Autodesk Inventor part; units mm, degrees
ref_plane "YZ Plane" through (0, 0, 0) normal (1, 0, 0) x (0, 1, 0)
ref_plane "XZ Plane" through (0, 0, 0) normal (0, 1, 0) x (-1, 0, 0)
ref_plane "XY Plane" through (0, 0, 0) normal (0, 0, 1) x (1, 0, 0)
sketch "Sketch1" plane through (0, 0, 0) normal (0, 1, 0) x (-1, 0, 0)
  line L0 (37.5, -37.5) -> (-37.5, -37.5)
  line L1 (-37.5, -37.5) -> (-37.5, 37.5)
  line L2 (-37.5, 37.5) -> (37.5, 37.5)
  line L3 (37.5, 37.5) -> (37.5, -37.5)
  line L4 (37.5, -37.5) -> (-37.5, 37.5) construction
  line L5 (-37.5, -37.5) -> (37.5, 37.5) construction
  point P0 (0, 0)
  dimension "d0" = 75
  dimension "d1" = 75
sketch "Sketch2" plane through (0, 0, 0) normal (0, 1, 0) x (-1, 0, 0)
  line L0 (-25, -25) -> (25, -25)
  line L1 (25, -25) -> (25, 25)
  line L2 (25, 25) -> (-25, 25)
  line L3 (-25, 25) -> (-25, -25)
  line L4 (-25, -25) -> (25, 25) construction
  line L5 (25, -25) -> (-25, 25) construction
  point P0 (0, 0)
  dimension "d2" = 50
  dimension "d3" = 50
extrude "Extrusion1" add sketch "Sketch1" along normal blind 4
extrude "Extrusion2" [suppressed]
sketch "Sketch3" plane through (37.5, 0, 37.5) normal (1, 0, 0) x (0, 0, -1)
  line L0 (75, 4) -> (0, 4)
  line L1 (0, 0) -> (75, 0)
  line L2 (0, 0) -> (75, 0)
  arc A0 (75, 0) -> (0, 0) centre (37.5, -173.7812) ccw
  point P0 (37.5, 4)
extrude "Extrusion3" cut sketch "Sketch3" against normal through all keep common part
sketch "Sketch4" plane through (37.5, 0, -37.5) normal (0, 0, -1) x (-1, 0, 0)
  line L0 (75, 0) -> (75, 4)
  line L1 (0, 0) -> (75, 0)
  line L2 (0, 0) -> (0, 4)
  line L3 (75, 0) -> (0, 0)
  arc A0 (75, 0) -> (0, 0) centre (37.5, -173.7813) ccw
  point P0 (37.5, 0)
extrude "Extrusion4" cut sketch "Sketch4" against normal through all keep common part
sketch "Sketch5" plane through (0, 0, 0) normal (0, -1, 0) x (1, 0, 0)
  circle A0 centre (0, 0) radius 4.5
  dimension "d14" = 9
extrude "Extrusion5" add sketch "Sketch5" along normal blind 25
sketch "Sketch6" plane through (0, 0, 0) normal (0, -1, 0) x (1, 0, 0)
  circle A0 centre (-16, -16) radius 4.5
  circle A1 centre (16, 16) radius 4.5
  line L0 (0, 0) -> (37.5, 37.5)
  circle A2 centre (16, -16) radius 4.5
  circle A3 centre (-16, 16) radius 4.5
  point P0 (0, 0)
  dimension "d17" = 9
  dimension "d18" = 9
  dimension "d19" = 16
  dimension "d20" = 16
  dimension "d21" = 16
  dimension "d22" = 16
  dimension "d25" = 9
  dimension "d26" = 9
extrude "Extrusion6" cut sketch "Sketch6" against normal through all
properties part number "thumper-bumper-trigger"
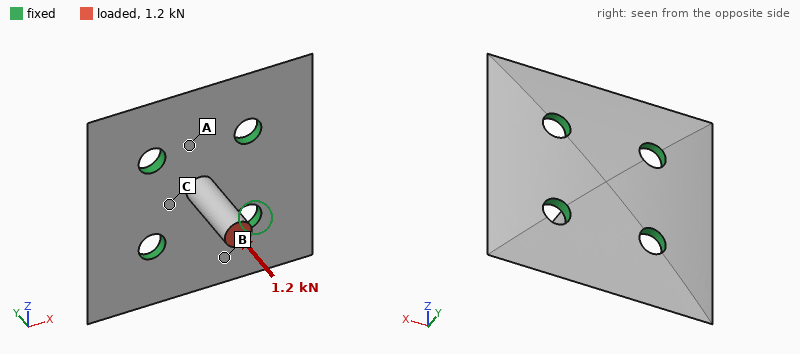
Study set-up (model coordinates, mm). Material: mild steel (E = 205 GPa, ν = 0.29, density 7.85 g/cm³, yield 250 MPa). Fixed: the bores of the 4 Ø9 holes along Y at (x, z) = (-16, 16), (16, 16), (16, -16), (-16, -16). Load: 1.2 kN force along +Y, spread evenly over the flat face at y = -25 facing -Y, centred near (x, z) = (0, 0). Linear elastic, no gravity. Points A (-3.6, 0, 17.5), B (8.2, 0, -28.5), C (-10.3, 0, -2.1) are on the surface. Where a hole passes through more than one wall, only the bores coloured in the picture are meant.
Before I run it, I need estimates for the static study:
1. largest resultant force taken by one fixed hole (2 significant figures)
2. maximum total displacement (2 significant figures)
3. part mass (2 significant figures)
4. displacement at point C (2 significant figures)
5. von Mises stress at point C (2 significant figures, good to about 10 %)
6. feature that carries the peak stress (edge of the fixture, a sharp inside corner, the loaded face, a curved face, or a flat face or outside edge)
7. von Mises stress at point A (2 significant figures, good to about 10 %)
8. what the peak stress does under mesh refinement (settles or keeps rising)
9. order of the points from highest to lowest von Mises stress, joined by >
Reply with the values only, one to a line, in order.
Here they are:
300 N
11 µm
95 g
5.1 µm
25 MPa
edge of the fixture
17 MPa
keeps rising
C > A > B
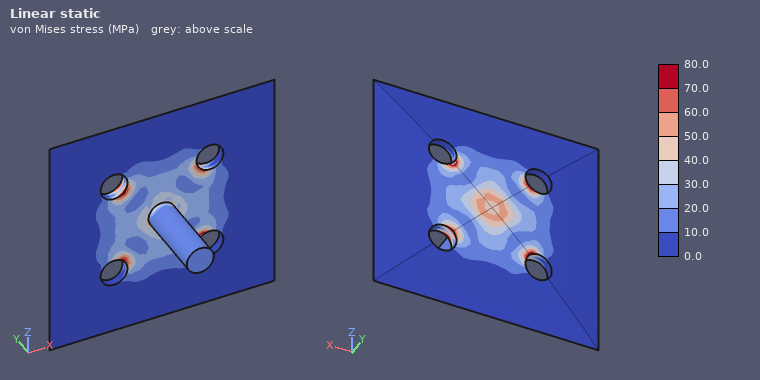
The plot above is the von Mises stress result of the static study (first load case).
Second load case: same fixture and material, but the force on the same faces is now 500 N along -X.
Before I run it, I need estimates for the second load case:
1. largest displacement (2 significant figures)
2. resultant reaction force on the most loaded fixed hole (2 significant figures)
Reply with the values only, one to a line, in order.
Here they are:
80 µm
320 N
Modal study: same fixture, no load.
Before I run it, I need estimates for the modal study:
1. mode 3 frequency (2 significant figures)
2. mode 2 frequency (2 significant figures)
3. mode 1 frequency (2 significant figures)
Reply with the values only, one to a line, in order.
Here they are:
6900 Hz
6500 Hz
6500 Hz
